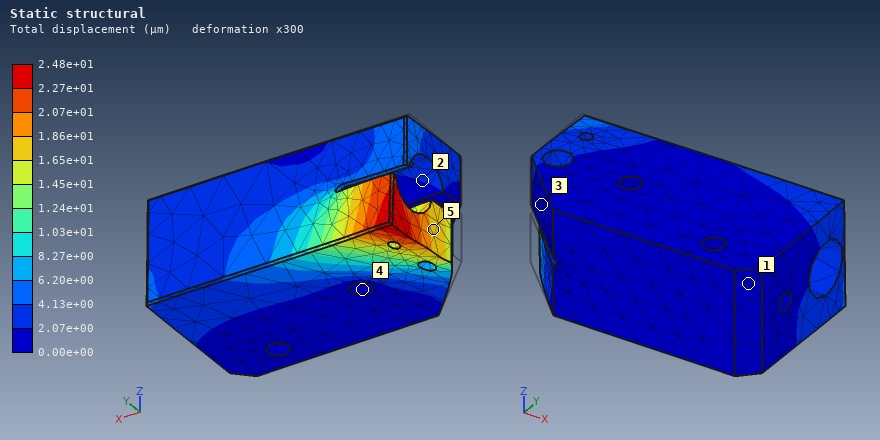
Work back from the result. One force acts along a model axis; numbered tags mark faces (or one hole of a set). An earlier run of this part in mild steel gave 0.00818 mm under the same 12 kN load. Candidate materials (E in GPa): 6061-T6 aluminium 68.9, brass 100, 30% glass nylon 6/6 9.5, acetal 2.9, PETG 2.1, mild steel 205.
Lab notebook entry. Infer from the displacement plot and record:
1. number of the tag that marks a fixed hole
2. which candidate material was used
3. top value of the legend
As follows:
4
6061-T6 aluminium
2.48e+01 µm
